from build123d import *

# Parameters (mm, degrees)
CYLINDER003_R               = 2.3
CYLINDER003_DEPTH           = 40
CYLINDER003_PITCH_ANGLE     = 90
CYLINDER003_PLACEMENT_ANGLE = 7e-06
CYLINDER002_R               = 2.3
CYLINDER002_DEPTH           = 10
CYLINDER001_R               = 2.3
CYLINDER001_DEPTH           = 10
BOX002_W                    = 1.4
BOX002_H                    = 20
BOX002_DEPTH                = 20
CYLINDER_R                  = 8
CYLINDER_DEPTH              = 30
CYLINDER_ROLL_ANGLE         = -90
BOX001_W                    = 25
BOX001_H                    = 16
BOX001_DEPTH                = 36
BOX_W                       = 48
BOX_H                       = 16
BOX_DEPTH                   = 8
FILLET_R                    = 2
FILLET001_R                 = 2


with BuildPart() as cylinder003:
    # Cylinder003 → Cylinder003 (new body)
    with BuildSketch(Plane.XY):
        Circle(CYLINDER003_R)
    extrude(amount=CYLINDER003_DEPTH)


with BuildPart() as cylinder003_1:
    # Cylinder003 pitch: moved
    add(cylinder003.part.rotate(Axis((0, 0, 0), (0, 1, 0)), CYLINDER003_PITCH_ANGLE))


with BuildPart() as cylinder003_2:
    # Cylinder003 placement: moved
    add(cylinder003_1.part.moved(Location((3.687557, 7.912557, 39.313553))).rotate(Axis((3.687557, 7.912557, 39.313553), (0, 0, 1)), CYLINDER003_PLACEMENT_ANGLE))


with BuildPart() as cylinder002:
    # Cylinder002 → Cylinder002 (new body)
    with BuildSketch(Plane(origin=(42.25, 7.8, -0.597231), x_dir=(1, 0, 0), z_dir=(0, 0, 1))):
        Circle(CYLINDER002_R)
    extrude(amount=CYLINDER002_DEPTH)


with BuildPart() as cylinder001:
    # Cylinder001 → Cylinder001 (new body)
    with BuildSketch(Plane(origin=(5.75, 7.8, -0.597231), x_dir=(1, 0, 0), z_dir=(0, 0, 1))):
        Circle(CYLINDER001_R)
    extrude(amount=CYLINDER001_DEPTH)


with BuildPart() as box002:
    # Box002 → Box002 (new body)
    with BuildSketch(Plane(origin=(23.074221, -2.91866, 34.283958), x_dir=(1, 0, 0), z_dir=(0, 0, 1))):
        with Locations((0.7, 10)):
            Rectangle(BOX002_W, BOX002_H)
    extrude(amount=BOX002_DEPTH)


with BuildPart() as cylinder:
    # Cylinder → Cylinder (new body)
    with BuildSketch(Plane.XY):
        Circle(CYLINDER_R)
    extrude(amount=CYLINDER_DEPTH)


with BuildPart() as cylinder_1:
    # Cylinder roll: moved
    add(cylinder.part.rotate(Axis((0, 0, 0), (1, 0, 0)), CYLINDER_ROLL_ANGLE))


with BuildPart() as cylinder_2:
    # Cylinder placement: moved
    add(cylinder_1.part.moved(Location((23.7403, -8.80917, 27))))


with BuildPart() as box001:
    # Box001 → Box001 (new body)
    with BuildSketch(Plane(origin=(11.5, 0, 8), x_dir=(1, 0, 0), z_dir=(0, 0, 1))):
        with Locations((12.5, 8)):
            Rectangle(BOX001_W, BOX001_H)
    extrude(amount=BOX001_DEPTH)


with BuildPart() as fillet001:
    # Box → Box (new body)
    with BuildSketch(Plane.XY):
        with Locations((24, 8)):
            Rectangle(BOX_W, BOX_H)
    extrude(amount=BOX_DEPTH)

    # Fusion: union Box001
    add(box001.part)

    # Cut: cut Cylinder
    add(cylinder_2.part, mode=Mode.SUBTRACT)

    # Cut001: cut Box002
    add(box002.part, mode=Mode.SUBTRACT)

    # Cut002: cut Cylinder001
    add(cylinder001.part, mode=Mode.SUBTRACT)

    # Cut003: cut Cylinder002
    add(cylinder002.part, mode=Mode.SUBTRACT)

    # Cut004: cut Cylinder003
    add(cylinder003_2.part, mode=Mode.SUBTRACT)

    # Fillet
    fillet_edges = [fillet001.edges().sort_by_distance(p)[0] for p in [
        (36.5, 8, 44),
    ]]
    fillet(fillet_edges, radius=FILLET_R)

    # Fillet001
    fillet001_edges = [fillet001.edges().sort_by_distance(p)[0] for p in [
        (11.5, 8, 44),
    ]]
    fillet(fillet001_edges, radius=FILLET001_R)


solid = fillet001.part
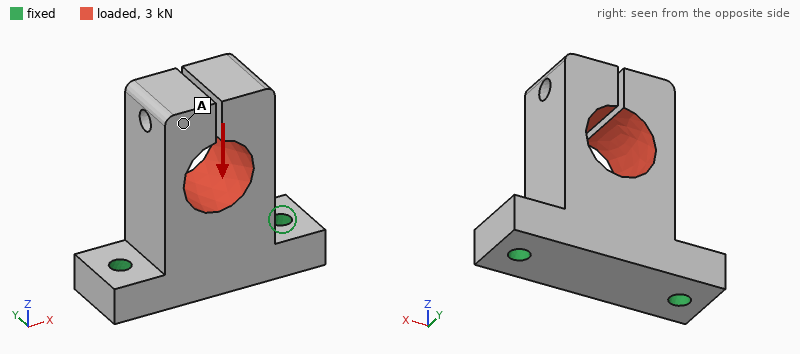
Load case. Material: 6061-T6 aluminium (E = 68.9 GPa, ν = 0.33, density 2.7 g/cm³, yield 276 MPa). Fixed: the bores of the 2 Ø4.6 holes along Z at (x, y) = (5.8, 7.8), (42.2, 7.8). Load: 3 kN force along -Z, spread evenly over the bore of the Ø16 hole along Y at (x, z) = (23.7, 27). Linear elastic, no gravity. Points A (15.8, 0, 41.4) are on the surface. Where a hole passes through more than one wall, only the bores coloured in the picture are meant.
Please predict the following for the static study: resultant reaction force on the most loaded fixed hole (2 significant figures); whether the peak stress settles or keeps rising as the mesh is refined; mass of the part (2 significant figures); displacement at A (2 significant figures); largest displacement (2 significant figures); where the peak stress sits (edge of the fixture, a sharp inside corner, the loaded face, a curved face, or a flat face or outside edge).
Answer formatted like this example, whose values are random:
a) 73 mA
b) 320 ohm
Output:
a) 1.6 kN
b) keeps rising
c) 44 g
d) 71 µm
e) 97 µm
f) edge of the fixture
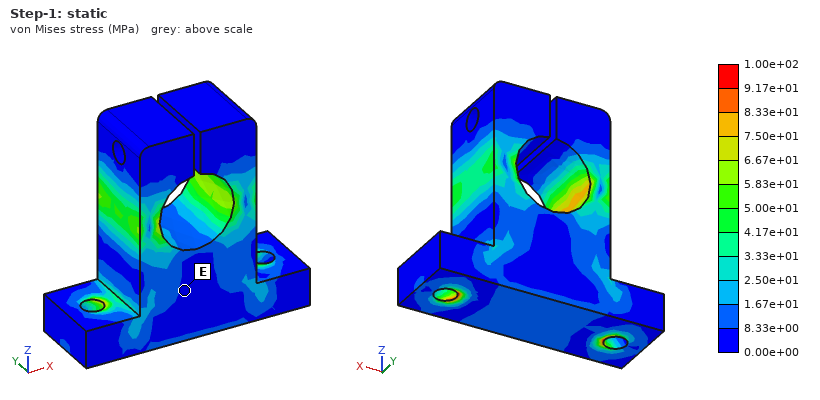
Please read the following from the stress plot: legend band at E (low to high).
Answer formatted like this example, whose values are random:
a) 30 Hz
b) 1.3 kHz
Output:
a) 0.00e+00 to 8.33e+00 MPa
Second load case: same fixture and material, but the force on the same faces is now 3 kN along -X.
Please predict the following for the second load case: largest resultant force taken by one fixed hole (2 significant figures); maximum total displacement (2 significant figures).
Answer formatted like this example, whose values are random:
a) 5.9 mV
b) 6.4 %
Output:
a) 2.7 kN
b) 0.18 mm
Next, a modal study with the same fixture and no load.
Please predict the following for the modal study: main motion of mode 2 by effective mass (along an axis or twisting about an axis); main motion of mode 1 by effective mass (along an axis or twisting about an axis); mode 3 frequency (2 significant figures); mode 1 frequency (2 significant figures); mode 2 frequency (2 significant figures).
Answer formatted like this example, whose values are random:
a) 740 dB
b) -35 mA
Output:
a) along X
b) along Y
c) 4600 Hz
d) 3900 Hz
e) 4200 Hz
